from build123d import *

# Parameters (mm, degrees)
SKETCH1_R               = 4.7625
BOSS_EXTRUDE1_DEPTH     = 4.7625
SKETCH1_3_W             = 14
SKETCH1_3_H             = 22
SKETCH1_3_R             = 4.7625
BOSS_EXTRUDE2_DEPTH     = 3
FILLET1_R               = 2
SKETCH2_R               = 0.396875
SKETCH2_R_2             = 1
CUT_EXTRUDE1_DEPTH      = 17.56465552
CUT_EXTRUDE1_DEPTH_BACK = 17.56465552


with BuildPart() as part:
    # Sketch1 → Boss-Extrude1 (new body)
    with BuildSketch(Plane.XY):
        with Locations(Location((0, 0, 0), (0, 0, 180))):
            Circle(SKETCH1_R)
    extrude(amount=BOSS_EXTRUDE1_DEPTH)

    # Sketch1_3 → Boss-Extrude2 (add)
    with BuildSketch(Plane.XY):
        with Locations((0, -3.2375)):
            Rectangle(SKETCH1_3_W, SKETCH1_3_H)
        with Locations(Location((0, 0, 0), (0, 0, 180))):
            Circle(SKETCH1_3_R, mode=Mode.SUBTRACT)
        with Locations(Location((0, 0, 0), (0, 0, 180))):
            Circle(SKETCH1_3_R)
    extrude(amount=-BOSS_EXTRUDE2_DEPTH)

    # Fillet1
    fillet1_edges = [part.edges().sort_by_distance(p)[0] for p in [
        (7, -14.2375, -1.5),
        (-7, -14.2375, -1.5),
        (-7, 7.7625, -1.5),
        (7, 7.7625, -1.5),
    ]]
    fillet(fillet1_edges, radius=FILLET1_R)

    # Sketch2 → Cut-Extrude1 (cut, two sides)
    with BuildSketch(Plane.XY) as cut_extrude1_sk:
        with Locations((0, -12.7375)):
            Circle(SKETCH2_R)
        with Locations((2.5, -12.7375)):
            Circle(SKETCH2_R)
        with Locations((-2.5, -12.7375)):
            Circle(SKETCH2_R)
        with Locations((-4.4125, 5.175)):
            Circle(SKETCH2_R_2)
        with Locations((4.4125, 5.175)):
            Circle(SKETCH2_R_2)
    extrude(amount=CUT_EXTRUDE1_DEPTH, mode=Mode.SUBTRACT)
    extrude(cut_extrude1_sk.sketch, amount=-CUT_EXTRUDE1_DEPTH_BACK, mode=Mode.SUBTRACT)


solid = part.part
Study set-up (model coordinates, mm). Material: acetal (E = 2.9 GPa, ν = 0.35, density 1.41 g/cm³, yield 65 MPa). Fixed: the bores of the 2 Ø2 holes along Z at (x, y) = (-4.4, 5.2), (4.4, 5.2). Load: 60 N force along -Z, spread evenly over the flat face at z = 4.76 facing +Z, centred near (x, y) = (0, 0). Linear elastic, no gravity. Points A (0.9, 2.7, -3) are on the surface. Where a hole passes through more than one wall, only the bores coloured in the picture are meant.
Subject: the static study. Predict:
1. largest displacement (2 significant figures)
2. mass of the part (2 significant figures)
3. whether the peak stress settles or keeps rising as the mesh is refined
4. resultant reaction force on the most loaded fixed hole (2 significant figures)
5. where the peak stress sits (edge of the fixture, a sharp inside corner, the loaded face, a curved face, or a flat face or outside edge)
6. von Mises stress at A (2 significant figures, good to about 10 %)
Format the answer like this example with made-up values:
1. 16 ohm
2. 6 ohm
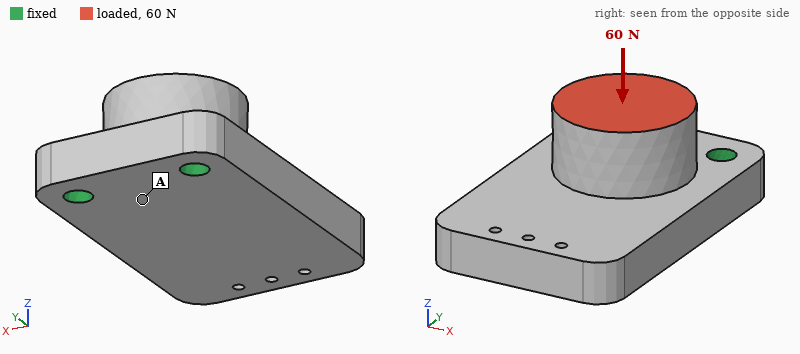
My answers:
1. 0.15 mm
2. 1.7 g
3. keeps rising
4. 30 N
5. edge of the fixture
6. 3.8 MPa
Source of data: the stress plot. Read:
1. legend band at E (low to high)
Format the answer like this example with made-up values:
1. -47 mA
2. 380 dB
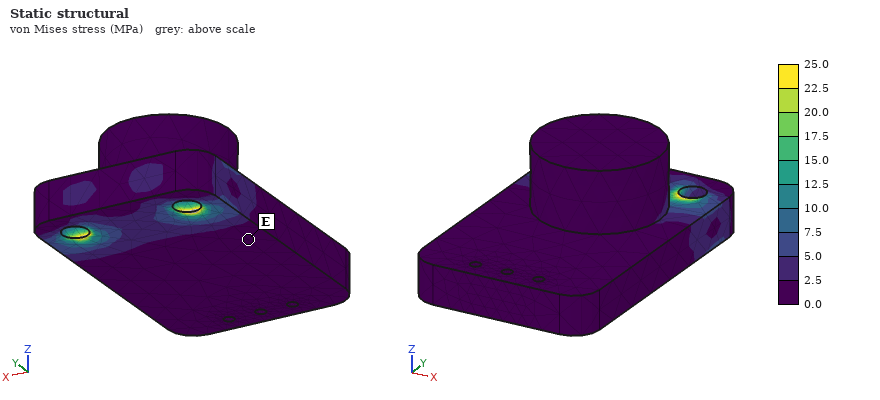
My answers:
1. 0.0 to 2.5 MPa
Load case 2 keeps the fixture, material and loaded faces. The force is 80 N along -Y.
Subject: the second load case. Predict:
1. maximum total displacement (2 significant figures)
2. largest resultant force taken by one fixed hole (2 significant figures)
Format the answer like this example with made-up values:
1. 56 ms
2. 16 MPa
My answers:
1. 0.31 mm
2. 42 N
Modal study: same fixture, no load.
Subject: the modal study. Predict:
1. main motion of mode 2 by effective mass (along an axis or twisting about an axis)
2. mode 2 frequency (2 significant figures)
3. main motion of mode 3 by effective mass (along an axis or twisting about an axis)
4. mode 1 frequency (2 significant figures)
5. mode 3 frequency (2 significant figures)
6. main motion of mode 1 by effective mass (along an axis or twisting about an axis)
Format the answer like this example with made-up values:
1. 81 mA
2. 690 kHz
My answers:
1. along X
2. 6400 Hz
3. along X
4. 2200 Hz
5. 7000 Hz
6. along Z
